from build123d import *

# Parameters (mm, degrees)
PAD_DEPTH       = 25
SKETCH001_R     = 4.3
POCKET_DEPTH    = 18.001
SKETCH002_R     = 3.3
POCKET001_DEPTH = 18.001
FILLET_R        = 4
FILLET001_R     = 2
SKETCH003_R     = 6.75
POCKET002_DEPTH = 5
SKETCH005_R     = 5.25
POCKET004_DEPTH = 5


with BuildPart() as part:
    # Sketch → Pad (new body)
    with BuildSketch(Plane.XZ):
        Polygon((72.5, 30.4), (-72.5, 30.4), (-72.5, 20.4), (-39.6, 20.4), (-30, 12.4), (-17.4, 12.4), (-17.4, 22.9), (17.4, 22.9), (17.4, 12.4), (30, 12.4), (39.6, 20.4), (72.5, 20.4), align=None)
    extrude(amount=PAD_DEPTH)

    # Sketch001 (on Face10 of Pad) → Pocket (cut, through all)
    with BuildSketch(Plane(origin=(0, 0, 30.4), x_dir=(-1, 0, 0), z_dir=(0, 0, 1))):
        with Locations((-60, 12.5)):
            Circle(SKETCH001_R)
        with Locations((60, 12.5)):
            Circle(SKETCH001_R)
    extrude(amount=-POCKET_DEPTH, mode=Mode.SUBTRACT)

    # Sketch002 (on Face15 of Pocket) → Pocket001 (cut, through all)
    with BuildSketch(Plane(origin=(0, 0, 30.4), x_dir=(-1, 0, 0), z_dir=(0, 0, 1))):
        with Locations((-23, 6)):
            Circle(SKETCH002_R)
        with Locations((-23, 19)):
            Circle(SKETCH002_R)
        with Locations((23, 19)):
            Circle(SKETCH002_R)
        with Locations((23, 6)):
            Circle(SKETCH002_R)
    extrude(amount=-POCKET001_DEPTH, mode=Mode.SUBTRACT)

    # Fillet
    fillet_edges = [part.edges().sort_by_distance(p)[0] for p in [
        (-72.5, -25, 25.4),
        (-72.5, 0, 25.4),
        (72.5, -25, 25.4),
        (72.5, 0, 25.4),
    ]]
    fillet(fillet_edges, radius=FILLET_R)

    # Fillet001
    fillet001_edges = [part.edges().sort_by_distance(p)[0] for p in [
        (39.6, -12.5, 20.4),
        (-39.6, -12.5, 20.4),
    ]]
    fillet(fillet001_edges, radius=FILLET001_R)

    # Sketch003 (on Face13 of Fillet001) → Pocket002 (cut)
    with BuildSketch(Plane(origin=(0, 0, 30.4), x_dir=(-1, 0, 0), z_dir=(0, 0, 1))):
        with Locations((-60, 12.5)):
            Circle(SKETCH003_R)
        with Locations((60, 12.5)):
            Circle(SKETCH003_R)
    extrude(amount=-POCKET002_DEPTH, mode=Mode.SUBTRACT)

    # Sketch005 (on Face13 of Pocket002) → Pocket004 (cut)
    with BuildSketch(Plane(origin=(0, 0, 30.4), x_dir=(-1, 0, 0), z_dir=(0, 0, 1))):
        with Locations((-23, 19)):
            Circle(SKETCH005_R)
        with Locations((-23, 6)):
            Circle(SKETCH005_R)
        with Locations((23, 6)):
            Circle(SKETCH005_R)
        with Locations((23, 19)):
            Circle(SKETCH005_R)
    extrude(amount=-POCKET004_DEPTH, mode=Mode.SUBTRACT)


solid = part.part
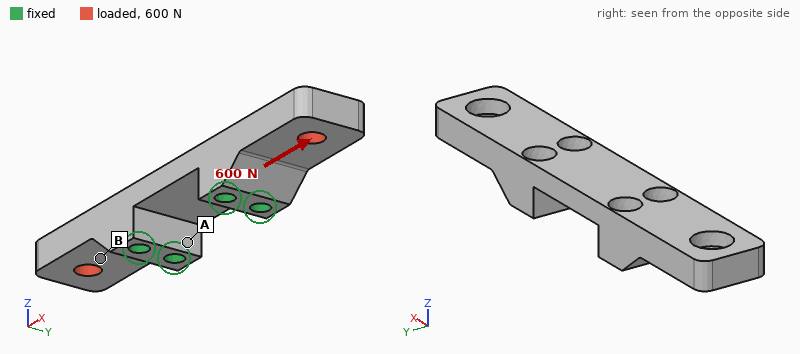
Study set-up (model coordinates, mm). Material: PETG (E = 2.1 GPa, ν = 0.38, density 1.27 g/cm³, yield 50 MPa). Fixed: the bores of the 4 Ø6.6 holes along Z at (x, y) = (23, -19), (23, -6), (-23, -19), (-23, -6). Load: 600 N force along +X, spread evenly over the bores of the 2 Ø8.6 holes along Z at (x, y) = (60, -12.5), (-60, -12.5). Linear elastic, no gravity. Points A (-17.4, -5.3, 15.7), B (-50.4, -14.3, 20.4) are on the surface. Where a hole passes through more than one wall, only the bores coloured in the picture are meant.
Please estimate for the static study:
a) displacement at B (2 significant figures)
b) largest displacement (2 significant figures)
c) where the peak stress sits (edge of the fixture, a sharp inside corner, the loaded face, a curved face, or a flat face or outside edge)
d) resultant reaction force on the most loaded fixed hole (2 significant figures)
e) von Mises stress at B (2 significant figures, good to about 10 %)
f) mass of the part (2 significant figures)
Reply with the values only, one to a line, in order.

26 µm
89 µm
the loaded face
150 N
3.1 MPa
45 g
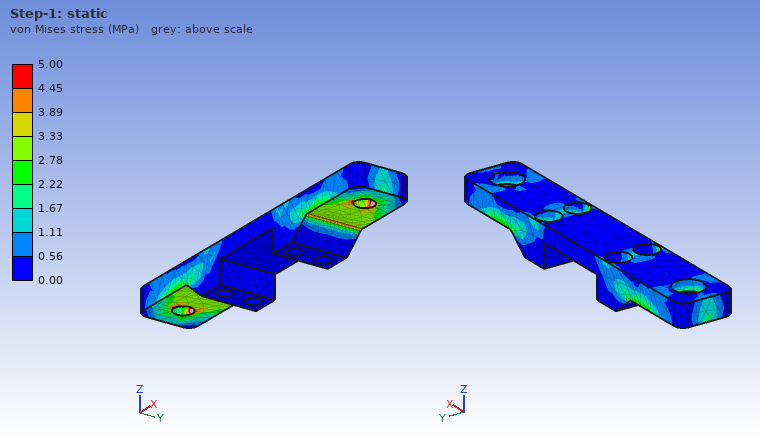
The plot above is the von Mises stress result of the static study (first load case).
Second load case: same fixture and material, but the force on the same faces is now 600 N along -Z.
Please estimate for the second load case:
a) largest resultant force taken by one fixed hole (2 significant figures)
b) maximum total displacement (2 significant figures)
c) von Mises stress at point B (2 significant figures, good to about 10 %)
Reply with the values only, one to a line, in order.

170 N
1.1 mm
7.6 MPa
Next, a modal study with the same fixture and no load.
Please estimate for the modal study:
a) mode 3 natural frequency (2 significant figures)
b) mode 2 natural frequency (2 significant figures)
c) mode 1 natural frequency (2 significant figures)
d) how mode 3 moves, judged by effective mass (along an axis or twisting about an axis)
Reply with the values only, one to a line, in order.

2000 Hz
1200 Hz
1200 Hz
along Y
